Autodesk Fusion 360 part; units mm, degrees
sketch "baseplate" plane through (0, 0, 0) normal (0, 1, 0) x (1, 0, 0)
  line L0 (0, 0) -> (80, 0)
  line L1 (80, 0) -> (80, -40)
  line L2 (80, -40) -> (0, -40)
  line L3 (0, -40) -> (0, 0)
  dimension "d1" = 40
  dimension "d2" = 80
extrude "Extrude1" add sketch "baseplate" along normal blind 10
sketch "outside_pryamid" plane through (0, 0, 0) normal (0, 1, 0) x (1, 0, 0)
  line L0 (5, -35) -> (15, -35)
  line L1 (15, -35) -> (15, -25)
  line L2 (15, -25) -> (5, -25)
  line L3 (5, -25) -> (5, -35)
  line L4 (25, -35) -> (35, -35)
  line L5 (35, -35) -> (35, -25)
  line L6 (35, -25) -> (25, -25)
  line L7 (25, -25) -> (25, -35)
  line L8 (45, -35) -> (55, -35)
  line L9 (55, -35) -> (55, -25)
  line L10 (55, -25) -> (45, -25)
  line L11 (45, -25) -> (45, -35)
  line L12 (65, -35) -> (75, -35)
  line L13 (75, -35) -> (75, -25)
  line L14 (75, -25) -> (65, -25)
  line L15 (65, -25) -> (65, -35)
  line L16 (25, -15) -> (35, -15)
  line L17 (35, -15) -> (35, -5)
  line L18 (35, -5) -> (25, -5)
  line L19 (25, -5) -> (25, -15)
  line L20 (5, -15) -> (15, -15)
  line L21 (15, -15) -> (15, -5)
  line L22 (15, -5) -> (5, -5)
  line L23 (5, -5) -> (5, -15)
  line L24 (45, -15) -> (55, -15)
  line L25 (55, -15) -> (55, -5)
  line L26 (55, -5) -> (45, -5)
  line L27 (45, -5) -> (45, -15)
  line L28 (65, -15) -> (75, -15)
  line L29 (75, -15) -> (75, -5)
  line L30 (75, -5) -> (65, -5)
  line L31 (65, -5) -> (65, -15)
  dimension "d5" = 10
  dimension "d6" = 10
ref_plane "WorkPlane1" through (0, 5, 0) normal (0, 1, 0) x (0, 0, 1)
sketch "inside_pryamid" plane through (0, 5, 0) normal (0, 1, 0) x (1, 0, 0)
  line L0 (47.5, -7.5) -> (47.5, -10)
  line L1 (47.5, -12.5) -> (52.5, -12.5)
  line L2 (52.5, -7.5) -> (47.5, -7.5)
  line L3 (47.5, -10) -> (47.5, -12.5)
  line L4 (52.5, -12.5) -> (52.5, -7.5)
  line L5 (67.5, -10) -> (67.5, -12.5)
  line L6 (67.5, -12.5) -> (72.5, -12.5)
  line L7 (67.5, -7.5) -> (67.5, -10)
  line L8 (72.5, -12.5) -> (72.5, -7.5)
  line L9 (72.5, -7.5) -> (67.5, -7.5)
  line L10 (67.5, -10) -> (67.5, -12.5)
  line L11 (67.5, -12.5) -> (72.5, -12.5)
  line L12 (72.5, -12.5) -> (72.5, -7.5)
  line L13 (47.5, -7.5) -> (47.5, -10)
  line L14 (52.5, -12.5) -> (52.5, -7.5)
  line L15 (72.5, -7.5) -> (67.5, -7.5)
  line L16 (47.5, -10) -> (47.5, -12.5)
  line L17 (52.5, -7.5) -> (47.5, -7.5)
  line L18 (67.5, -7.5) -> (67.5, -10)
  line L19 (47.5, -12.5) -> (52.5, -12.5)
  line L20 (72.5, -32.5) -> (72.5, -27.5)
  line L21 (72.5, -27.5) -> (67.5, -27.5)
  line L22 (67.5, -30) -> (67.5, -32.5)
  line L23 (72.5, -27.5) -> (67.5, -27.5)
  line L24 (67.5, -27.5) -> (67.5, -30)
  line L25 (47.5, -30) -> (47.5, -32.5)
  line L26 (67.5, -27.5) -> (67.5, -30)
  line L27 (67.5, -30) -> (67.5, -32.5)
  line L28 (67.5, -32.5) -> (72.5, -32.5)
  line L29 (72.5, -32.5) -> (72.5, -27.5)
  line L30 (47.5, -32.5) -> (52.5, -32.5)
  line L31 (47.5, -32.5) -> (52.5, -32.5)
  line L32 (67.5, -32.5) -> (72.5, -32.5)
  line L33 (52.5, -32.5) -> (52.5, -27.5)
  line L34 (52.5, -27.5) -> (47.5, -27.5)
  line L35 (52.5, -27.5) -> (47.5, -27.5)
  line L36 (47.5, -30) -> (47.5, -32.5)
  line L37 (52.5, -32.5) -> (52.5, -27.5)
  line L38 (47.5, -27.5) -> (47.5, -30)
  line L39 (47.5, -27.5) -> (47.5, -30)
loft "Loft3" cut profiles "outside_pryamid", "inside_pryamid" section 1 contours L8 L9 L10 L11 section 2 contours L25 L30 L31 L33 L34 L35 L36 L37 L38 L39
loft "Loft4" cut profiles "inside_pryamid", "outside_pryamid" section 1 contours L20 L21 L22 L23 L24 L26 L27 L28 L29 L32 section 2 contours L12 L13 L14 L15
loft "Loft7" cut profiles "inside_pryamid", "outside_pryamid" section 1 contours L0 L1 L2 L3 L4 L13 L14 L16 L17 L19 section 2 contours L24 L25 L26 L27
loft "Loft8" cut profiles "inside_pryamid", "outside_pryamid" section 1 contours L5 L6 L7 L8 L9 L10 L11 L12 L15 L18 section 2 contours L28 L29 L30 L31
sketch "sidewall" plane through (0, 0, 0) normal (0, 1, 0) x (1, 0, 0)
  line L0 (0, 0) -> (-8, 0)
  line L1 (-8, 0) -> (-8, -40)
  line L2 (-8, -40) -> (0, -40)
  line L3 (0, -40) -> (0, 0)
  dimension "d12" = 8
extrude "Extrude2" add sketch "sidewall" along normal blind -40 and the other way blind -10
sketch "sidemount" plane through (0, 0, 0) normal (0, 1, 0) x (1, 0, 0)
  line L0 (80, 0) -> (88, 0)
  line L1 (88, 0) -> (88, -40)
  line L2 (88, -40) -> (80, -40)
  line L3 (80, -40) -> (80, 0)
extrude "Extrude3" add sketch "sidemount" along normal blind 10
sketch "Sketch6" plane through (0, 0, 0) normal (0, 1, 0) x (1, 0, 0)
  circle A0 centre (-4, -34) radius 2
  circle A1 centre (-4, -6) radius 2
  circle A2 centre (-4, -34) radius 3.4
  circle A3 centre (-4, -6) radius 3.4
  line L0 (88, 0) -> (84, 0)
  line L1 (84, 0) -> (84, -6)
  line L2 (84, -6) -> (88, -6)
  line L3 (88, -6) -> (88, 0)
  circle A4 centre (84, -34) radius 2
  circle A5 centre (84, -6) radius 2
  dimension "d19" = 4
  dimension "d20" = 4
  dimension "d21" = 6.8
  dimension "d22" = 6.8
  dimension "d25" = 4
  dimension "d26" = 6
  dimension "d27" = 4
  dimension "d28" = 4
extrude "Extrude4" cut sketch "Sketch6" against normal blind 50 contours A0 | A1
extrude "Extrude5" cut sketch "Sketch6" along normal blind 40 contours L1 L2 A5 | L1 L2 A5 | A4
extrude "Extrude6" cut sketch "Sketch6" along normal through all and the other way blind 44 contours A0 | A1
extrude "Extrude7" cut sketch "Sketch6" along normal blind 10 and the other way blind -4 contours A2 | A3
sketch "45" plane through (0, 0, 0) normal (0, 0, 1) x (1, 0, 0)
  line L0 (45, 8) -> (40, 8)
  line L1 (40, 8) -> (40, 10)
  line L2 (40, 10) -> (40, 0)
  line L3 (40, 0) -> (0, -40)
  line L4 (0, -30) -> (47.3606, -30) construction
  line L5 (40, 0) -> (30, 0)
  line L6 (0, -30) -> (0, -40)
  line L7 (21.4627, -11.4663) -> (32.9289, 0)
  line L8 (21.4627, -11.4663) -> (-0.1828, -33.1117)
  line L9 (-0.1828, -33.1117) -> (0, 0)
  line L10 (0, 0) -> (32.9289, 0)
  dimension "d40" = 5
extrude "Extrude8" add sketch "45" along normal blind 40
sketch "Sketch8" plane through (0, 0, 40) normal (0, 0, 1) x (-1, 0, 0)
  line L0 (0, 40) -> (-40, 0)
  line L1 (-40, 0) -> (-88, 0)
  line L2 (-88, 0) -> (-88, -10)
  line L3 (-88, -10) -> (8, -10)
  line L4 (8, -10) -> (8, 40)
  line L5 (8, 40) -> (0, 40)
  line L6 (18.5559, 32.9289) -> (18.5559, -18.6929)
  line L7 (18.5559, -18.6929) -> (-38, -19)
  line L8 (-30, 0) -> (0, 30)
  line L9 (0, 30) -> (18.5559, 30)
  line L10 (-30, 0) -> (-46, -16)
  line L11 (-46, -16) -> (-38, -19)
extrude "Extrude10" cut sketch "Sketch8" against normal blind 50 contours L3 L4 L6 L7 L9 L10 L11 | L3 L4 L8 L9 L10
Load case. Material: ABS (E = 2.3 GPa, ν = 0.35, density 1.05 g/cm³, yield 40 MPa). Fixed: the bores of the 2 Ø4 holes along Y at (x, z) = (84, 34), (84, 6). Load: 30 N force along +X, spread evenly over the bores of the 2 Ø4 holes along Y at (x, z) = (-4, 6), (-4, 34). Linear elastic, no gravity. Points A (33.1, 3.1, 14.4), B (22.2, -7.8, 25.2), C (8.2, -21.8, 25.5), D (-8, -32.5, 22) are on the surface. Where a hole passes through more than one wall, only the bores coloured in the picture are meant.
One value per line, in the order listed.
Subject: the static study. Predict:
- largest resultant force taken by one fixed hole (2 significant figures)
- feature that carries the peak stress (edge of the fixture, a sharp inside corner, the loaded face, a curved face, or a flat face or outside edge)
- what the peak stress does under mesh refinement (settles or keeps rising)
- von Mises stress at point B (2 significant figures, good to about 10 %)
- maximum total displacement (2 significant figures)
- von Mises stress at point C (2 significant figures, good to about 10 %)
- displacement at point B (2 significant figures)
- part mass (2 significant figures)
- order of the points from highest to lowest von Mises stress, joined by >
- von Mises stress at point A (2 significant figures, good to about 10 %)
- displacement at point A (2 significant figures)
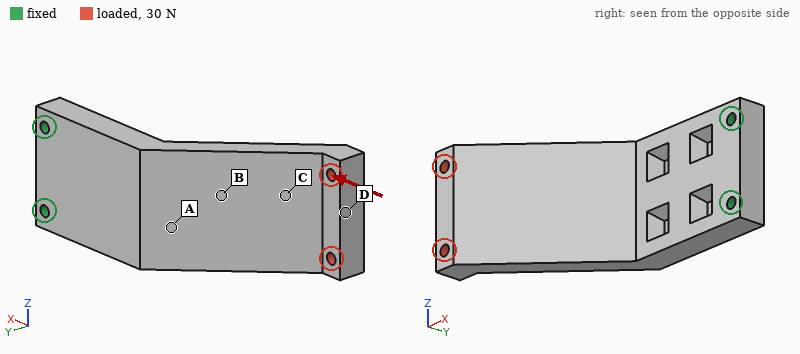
15 N
edge of the fixture
keeps rising
2.0 MPa
1.3 mm
0.88 MPa
0.47 mm
39 g
A > B > C > D
2.7 MPa
0.28 mm
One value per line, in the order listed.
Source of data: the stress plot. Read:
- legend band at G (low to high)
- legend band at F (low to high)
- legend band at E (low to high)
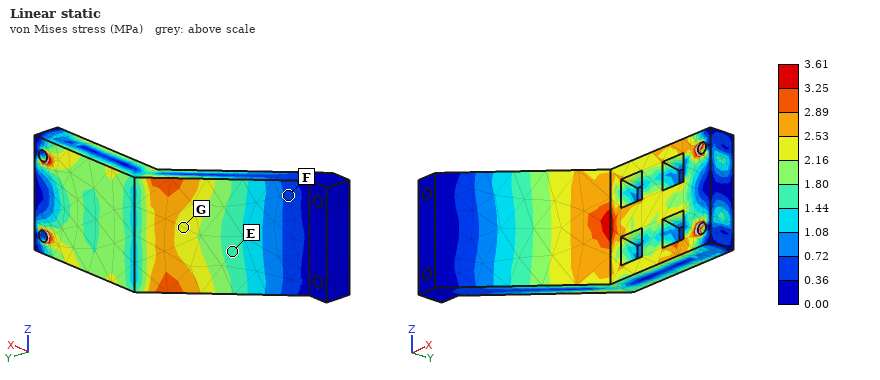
2.16 to 2.53 MPa
0.36 to 0.72 MPa
1.44 to 1.80 MPa
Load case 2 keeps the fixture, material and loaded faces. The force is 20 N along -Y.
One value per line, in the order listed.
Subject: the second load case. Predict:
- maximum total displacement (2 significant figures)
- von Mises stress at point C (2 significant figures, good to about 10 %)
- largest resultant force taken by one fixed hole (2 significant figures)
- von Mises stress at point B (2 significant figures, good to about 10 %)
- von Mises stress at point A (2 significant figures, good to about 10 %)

1.3 mm
0.90 MPa
10 N
1.6 MPa
2.1 MPa
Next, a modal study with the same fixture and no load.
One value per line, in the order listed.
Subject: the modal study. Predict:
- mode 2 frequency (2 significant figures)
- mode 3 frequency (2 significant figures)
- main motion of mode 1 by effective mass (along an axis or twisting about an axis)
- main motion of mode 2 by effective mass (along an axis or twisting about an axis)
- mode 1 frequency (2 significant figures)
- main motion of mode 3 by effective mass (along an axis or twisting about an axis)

490 Hz
810 Hz
along Y
along Z
200 Hz
along Y
